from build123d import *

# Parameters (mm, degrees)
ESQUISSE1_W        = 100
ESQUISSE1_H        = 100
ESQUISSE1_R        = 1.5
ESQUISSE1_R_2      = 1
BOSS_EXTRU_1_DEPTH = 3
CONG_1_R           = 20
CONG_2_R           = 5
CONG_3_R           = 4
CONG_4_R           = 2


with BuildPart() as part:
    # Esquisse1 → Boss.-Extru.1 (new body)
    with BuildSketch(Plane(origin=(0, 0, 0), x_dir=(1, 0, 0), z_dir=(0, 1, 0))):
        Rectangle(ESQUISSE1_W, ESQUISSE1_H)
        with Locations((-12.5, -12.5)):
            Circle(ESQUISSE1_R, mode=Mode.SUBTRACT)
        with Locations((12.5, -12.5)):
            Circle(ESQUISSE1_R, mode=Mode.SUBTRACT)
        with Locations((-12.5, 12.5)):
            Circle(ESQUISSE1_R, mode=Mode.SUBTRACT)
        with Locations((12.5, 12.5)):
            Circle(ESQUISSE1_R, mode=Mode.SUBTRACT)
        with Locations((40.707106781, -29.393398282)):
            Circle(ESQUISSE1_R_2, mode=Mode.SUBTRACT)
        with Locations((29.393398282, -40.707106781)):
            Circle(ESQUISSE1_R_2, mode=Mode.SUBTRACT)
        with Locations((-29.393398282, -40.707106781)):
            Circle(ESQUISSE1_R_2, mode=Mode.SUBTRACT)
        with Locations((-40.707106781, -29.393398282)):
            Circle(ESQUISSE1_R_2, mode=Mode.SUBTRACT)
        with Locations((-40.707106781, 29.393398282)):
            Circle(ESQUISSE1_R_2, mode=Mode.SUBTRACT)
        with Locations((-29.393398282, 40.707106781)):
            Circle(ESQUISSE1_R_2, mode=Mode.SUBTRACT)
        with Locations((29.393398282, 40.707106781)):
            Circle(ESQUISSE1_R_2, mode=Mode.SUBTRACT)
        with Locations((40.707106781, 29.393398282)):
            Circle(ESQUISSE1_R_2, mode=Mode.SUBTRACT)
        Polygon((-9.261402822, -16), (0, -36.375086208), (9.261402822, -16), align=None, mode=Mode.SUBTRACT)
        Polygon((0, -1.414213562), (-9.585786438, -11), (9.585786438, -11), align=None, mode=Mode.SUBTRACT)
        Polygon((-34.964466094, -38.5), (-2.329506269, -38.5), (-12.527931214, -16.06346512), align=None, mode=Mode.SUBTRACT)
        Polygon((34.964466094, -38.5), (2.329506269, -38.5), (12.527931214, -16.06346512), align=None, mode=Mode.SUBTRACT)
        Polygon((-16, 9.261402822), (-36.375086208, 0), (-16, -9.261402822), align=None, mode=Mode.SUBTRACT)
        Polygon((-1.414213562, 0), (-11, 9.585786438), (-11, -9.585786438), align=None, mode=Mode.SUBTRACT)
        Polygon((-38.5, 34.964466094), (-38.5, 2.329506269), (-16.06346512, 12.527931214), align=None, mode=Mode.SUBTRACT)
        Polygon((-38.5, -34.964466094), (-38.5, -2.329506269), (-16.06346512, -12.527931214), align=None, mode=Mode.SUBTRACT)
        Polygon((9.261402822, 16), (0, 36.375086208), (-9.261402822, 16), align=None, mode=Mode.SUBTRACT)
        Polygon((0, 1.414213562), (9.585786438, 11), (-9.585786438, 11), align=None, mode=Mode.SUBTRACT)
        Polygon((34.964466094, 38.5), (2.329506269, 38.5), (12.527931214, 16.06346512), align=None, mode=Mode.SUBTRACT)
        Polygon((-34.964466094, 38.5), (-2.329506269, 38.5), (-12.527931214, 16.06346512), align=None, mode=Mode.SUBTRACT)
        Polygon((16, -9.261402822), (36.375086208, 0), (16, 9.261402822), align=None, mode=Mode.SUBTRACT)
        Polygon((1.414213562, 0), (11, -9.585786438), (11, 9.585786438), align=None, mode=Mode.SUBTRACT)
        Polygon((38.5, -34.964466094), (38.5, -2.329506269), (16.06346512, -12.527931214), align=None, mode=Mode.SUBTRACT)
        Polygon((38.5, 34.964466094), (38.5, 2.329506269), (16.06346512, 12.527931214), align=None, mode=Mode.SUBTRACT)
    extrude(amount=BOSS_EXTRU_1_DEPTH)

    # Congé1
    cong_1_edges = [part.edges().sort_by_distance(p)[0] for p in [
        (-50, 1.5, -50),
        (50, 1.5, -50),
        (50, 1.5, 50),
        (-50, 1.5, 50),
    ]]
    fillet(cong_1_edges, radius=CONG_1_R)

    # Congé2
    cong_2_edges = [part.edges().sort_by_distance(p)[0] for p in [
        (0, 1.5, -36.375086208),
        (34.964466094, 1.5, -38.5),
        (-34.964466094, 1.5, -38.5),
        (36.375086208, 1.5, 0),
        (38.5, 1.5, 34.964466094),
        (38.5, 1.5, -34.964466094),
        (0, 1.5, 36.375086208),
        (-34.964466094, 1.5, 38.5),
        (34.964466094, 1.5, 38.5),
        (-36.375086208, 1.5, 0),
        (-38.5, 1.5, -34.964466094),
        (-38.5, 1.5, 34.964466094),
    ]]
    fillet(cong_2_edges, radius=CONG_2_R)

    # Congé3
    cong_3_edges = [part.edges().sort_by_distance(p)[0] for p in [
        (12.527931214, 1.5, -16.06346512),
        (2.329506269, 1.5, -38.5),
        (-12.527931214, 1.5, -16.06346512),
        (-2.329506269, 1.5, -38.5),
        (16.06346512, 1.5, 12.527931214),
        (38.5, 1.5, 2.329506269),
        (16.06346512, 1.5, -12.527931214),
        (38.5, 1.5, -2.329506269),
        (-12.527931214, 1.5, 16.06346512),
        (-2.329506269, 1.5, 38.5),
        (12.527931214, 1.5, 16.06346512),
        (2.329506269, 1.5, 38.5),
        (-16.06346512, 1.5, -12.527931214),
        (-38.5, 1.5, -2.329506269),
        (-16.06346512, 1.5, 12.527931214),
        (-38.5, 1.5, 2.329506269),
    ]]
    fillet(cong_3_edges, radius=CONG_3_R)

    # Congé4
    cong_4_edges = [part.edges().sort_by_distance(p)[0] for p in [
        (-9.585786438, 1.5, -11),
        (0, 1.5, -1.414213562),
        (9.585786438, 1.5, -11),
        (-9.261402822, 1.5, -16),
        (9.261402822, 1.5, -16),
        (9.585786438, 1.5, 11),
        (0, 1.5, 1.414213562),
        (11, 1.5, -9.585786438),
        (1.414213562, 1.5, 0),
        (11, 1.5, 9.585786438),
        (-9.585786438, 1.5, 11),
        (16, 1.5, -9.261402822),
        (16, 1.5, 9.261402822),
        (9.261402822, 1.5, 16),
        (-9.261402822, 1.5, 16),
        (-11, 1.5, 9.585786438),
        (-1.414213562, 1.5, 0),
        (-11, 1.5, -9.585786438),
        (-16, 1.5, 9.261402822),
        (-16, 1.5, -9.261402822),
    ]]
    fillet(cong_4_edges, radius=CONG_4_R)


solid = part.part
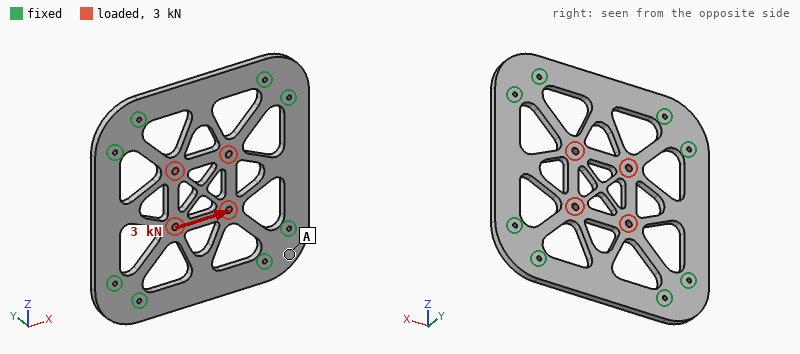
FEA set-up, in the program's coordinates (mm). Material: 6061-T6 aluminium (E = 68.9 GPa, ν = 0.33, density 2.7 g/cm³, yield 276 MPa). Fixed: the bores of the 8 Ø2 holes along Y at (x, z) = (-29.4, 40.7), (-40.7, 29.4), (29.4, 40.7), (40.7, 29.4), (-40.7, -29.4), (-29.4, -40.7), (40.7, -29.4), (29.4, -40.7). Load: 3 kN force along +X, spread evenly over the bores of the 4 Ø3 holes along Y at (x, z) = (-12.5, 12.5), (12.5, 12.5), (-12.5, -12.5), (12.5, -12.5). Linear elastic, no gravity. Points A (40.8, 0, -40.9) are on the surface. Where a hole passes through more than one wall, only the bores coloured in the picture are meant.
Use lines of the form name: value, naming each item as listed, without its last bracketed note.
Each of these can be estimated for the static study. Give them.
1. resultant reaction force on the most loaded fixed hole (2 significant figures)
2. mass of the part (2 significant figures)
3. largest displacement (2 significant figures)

resultant reaction force on the most loaded fixed hole: 540 N
mass of the part: 49 g
largest displacement: 26 µm
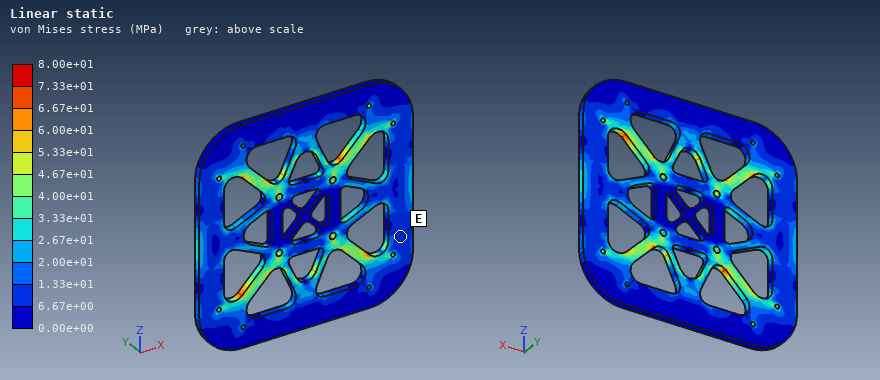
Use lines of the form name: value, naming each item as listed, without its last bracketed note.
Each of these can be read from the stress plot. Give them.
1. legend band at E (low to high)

legend band at E: 6.67e+00 to 1.33e+01 MPa
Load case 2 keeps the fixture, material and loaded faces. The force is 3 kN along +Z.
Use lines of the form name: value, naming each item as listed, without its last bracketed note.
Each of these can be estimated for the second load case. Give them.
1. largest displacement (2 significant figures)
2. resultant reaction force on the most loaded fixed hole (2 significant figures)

largest displacement: 26 µm
resultant reaction force on the most loaded fixed hole: 540 N
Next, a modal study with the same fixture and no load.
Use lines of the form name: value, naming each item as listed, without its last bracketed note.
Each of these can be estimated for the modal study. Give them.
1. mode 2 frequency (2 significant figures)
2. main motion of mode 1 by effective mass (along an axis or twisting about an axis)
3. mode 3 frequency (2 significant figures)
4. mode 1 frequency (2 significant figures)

mode 2 frequency: 3700 Hz
main motion of mode 1 by effective mass: along Y
mode 3 frequency: 3700 Hz
mode 1 frequency: 2000 Hz
